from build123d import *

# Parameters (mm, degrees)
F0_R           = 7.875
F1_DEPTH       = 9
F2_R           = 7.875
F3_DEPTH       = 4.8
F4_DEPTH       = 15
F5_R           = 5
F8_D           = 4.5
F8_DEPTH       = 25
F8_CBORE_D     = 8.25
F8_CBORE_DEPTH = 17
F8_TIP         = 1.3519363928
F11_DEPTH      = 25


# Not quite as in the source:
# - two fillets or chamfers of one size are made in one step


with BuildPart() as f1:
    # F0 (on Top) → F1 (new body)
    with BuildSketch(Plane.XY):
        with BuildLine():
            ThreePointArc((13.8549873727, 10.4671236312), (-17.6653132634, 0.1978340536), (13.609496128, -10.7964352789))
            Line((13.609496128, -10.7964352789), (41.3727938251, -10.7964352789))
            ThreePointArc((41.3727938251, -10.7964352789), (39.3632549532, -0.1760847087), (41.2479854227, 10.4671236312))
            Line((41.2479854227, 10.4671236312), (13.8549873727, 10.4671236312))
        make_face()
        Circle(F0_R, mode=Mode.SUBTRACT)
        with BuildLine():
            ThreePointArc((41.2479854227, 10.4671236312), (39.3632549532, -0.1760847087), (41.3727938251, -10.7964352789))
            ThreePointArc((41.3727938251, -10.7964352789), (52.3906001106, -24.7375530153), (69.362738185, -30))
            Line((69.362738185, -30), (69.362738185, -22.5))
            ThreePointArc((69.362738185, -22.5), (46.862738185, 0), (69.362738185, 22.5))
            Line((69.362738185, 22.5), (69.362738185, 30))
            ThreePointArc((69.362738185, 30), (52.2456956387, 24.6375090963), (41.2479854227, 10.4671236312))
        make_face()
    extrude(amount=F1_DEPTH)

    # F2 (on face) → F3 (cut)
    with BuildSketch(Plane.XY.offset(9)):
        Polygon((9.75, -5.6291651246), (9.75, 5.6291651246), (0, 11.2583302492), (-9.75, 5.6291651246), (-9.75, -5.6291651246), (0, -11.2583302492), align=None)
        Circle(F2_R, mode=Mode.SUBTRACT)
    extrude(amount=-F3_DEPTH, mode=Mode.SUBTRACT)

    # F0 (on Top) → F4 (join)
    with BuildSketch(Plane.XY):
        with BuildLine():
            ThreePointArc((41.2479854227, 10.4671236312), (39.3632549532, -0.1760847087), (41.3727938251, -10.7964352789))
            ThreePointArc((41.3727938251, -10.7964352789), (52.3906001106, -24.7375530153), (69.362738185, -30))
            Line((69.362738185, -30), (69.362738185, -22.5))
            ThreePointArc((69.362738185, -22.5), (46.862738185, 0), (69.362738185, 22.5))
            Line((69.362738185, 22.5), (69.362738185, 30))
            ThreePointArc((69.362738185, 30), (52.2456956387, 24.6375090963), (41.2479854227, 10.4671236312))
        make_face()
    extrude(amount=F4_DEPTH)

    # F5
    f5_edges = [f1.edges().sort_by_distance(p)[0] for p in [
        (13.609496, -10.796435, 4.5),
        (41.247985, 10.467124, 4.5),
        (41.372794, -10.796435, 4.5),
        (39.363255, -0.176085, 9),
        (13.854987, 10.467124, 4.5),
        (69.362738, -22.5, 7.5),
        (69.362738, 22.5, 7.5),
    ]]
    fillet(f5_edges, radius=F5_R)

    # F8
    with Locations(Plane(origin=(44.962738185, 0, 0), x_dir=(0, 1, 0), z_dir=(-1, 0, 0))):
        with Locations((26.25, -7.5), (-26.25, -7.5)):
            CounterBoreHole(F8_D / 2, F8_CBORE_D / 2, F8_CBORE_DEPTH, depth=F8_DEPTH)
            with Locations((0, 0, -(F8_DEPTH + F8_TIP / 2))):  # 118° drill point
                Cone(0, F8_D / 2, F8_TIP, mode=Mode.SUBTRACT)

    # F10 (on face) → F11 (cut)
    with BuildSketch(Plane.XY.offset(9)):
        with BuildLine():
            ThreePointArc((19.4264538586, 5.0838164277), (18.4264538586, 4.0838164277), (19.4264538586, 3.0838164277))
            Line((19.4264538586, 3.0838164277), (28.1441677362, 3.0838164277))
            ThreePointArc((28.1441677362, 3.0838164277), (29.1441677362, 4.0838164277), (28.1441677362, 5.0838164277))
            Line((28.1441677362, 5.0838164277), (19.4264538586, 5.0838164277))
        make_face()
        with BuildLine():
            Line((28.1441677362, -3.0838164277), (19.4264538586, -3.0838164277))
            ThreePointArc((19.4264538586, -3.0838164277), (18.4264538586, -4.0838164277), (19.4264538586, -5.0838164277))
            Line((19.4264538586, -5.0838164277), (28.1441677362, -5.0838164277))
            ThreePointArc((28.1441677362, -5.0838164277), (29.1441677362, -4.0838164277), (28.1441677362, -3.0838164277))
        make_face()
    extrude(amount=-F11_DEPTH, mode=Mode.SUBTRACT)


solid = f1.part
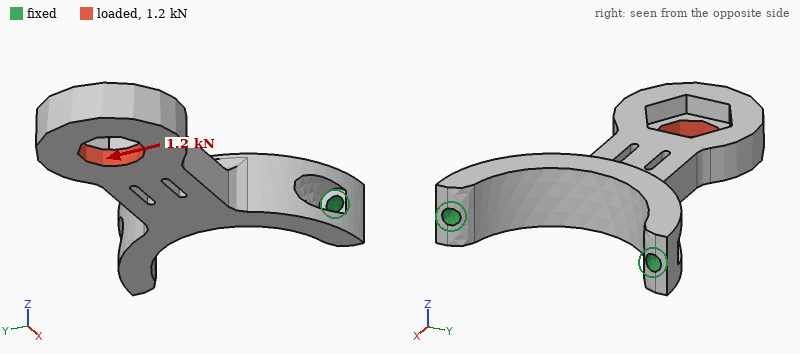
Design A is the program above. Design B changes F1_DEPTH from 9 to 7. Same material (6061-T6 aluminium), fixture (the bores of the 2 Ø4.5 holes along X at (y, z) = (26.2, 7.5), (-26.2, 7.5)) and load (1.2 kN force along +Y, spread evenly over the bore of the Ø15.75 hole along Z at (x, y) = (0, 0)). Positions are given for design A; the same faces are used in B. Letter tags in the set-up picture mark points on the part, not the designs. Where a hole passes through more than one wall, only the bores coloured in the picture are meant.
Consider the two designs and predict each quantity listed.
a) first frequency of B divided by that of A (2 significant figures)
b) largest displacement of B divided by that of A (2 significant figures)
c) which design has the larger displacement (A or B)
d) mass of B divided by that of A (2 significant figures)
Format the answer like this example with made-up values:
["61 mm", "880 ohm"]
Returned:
["0.98", "1.2", "B", "0.88"]
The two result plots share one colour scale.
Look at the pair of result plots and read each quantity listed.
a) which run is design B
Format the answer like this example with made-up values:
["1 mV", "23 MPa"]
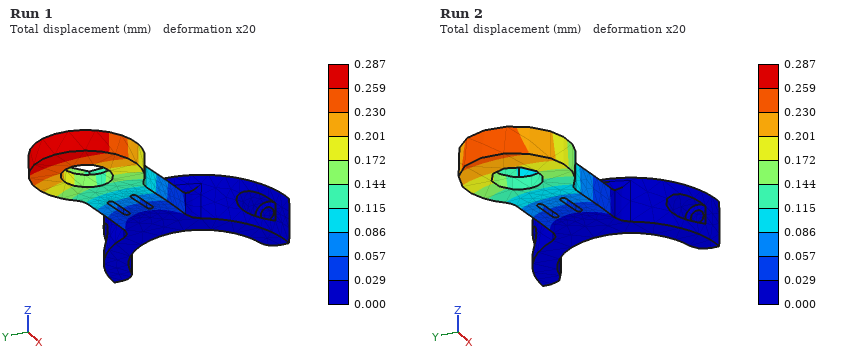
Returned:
["Run 1"]
